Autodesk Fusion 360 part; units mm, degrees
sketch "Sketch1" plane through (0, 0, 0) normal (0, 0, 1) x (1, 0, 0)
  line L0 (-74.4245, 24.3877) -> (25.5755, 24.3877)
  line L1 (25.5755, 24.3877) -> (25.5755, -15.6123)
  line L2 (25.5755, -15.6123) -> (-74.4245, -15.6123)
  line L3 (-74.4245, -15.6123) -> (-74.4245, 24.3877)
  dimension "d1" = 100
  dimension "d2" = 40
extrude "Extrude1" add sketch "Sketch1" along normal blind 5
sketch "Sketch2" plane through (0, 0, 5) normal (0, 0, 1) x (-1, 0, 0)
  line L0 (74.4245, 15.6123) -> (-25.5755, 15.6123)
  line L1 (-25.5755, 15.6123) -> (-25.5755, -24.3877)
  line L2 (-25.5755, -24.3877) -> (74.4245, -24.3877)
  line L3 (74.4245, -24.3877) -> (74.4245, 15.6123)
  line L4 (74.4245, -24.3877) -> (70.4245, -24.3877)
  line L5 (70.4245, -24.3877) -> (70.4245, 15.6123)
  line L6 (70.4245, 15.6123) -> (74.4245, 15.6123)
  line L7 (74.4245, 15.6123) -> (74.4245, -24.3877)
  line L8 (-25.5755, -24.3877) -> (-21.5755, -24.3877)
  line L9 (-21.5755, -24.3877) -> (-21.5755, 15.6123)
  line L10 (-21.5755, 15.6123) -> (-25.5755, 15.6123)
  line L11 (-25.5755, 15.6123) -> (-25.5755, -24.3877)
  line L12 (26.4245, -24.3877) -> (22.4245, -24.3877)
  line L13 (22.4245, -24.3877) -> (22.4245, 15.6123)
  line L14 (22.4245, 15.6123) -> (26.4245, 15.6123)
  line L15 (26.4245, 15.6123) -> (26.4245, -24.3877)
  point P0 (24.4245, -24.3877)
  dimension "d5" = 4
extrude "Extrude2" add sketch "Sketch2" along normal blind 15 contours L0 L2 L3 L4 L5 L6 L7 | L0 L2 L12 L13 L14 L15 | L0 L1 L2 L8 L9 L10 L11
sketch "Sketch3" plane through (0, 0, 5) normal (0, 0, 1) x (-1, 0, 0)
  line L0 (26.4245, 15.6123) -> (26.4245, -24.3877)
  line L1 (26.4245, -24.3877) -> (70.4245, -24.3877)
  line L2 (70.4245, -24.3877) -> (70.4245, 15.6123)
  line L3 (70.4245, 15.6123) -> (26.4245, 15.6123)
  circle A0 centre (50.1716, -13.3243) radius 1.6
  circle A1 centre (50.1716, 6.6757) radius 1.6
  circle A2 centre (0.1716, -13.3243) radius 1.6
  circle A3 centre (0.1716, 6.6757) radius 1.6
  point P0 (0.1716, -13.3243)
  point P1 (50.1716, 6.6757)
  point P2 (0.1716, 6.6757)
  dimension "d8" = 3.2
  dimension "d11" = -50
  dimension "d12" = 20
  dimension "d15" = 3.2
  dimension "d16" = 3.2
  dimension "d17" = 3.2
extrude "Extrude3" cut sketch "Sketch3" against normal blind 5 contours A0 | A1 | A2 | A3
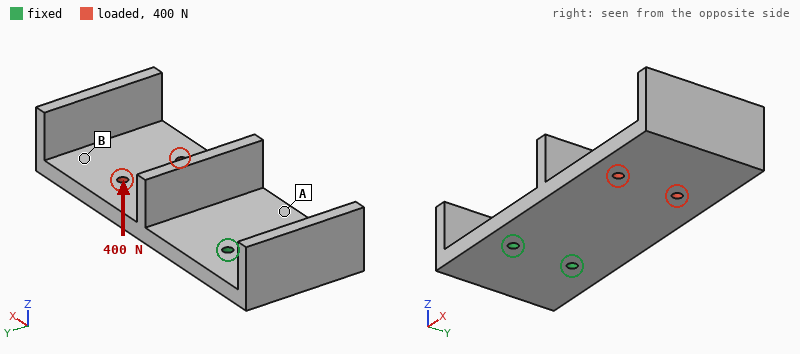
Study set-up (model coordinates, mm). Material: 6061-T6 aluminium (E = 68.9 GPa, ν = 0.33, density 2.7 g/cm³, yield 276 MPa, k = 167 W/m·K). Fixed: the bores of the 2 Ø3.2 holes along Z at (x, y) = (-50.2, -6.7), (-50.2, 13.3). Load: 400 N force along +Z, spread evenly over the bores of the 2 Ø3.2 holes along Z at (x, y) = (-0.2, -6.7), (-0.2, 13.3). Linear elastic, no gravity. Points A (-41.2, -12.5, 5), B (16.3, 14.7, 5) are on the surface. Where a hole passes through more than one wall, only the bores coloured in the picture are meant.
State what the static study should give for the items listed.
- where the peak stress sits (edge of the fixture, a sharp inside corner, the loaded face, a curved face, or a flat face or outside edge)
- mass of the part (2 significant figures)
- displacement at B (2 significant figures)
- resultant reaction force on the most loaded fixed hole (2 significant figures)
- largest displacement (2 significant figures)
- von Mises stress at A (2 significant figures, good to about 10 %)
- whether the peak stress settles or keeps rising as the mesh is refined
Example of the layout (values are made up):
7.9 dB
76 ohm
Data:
edge of the fixture
73 g
0.87 mm
200 N
1.1 mm
97 MPa
keeps rising
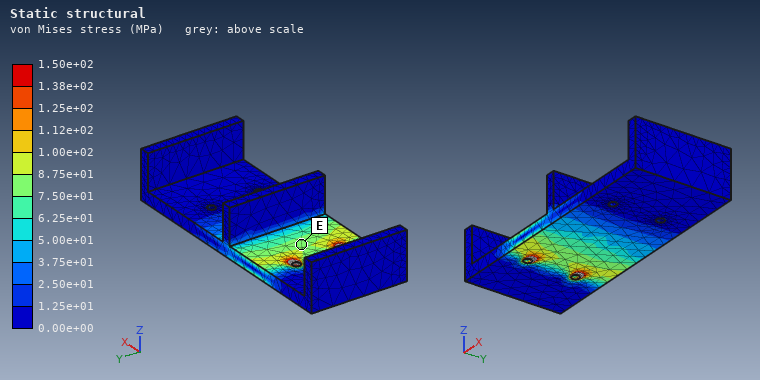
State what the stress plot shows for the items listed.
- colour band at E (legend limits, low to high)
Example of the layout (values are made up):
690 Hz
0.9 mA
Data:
7.50e+01 to 8.75e+01 MPa
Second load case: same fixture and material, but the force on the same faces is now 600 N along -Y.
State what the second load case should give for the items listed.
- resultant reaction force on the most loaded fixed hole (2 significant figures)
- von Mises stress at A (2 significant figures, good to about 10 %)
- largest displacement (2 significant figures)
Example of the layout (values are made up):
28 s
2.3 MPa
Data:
1.4 kN
15 MPa
44 µm
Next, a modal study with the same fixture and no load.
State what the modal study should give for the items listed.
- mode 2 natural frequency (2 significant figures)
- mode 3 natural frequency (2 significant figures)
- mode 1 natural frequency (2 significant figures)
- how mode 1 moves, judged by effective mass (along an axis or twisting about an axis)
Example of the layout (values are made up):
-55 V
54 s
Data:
2100 Hz
3000 Hz
560 Hz
along Z
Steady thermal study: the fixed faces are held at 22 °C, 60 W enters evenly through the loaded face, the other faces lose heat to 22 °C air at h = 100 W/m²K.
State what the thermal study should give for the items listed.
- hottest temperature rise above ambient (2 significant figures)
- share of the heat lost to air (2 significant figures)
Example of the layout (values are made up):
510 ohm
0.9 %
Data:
58 K
53 %
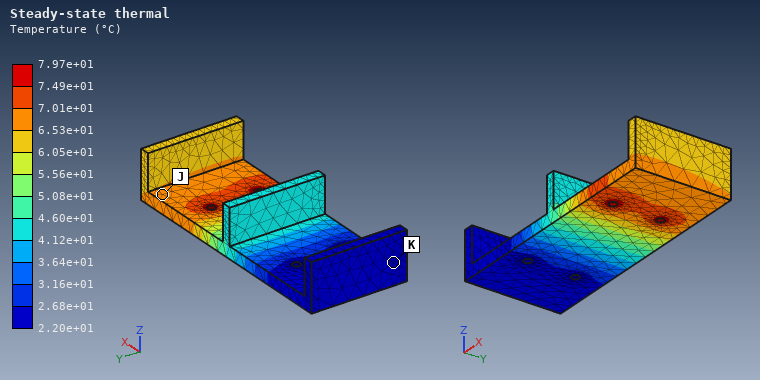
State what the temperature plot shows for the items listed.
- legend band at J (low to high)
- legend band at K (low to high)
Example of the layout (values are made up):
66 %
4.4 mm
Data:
6.53e+01 to 7.01e+01 °C
2.20e+01 to 2.68e+01 °C
